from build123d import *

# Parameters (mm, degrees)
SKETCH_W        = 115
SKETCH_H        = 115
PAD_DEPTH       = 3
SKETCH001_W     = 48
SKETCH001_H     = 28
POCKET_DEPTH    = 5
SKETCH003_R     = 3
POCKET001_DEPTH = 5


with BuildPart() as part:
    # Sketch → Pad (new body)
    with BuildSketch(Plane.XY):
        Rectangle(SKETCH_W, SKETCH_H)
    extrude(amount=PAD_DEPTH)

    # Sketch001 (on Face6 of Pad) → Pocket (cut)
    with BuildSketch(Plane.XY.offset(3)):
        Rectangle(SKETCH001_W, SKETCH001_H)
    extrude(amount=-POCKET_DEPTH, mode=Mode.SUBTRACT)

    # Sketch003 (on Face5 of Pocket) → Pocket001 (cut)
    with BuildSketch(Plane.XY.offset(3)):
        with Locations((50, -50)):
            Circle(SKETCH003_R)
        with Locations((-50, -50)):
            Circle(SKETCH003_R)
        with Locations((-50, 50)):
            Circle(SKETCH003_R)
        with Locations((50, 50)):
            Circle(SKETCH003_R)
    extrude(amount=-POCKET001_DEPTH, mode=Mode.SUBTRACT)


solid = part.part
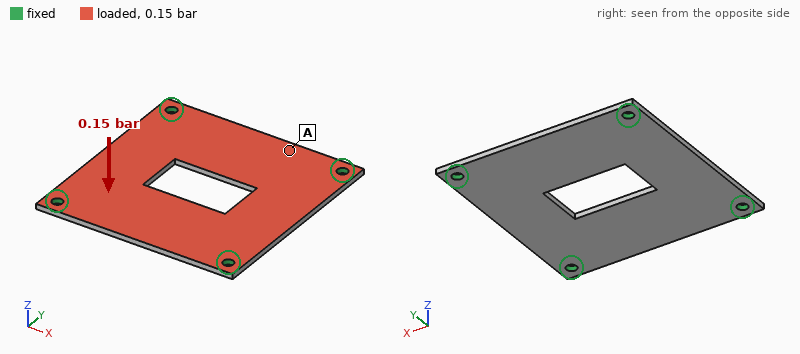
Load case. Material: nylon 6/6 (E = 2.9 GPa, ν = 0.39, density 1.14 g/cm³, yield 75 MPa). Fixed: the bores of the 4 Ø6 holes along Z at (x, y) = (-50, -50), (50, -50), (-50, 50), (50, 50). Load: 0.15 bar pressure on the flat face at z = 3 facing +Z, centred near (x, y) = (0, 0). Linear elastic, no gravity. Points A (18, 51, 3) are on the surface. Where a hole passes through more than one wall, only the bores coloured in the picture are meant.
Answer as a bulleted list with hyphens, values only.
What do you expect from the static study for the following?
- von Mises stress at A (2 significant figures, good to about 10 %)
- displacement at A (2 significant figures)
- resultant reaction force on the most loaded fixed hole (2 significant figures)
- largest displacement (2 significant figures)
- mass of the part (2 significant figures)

- 3.0 MPa
- 0.51 mm
- 44 N
- 1.7 mm
- 40 g
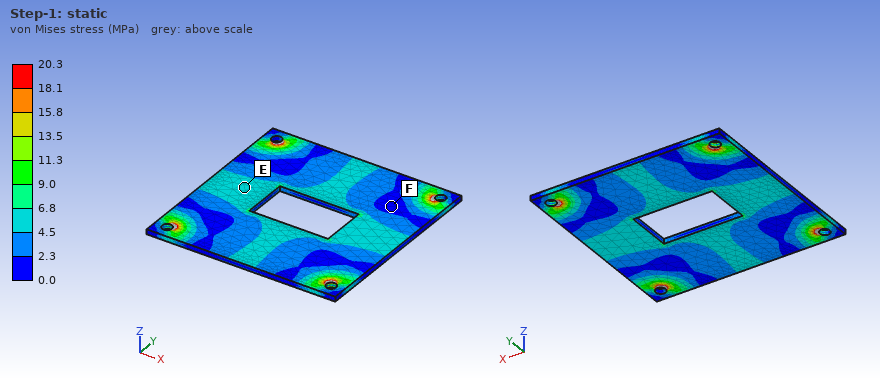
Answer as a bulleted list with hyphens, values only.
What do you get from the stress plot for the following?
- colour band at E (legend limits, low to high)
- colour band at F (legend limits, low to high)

- 4.5 to 6.8 MPa
- 0.0 to 2.3 MPa
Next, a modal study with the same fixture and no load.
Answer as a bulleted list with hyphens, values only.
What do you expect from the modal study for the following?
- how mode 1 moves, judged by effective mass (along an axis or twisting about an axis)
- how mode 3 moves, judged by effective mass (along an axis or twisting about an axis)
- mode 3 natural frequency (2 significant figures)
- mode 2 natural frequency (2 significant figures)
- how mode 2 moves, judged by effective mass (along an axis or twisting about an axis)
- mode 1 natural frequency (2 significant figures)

- along Z
- twisting about Y
- 560 Hz
- 530 Hz
- twisting about X
- 340 Hz
